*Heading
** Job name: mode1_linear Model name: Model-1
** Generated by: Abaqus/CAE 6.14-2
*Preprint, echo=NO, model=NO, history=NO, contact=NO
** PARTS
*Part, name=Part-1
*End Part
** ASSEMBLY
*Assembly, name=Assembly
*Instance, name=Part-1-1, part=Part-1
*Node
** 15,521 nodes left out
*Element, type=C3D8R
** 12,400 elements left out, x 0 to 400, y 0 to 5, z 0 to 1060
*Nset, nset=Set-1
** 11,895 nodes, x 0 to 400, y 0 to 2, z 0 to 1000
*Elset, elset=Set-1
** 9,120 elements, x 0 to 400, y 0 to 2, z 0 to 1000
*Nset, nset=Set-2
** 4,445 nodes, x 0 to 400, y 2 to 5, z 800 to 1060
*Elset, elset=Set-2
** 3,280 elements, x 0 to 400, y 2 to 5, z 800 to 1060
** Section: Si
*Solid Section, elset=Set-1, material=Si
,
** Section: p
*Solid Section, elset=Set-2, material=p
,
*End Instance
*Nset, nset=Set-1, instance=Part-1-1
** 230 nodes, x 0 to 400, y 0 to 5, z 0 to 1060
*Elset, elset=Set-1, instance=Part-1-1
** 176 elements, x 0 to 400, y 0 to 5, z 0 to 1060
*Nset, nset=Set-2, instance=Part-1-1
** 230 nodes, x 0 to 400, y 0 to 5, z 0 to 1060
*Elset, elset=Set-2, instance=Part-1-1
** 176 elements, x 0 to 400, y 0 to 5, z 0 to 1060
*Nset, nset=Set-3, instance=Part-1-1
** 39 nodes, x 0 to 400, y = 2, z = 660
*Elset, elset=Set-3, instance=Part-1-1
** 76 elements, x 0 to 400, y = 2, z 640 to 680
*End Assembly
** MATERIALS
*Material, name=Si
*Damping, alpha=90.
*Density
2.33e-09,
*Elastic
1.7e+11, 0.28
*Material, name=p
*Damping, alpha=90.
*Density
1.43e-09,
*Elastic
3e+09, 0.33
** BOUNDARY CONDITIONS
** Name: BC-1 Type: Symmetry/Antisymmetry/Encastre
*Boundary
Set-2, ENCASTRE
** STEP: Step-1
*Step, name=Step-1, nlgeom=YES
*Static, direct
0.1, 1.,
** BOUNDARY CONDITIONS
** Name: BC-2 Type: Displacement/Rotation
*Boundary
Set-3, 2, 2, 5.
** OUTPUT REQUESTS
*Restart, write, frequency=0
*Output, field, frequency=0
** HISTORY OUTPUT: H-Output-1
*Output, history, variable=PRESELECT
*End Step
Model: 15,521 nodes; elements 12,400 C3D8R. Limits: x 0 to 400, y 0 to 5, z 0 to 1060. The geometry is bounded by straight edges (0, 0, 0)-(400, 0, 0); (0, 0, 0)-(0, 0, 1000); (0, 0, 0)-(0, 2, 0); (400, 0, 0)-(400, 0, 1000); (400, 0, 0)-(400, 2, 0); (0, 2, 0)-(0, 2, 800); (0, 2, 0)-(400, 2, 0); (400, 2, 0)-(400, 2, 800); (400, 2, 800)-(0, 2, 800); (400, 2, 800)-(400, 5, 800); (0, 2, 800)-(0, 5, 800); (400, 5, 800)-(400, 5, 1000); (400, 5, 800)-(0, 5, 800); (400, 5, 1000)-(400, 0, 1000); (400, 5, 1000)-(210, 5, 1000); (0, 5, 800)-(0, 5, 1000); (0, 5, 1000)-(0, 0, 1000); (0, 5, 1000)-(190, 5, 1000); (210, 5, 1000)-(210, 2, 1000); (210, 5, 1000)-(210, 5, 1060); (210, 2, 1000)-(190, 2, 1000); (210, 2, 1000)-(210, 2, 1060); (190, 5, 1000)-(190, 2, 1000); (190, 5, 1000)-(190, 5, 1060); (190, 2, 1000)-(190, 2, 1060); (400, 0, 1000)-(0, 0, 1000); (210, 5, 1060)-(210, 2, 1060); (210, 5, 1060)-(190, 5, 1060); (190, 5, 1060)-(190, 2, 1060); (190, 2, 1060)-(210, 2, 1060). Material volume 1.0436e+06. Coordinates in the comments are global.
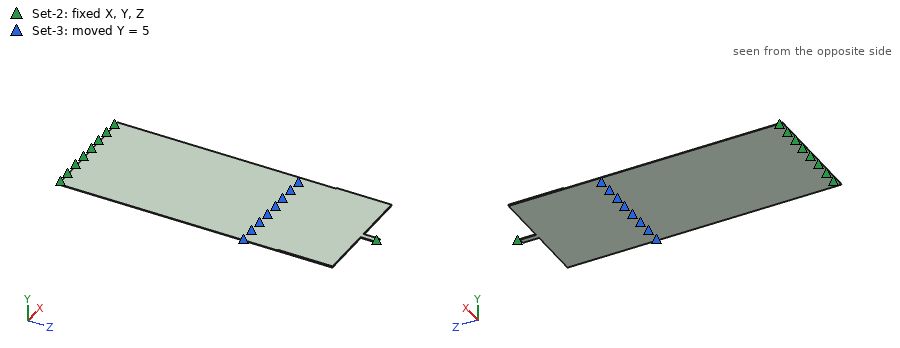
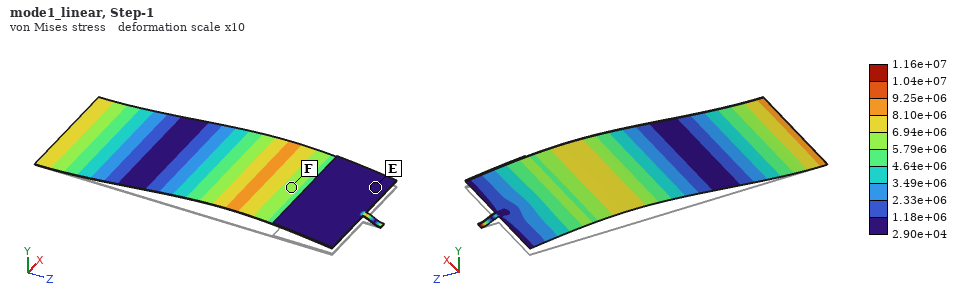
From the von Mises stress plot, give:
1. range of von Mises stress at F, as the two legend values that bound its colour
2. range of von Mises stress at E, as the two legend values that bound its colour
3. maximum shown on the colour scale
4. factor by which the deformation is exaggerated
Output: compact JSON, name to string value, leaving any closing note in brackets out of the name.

{"range of von Mises stress at F, as the two legend values that bound its colour": "5.79e+06 to 6.94e+06", "range of von Mises stress at E, as the two legend values that bound its colour": "2.90e+04 to 1.18e+06", "maximum shown on the colour scale": "1.16e+07", "factor by which the deformation is exaggerated": "10"}
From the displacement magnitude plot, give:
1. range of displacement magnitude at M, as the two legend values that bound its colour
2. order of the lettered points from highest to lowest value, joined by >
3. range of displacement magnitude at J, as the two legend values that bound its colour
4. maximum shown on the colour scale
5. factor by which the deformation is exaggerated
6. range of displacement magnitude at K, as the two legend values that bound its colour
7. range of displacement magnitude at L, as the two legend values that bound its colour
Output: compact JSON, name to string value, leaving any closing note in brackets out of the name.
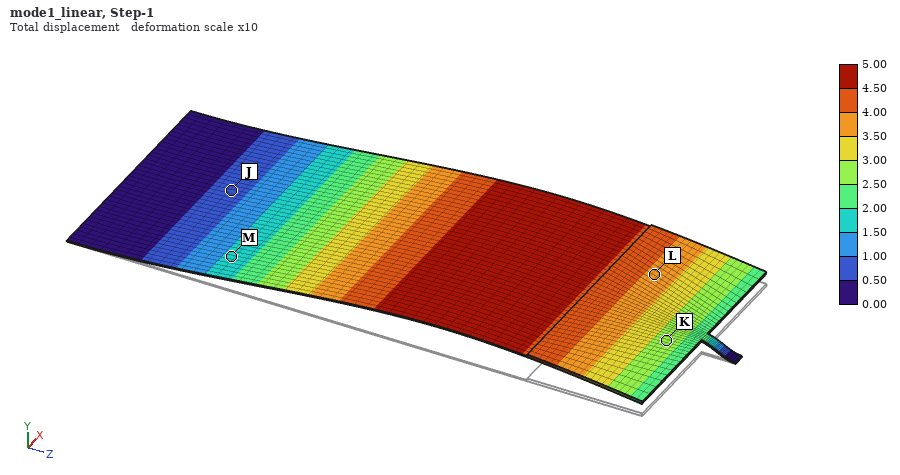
{"range of displacement magnitude at M, as the two legend values that bound its colour": "1.50 to 2.00", "order of the lettered points from highest to lowest value, joined by >": "L > K > M > J", "range of displacement magnitude at J, as the two legend values that bound its colour": "0.50 to 1.00", "maximum shown on the colour scale": "5.00", "factor by which the deformation is exaggerated": "10", "range of displacement magnitude at K, as the two legend values that bound its colour": "2.50 to 3.00", "range of displacement magnitude at L, as the two legend values that bound its colour": "3.50 to 4.00"}
